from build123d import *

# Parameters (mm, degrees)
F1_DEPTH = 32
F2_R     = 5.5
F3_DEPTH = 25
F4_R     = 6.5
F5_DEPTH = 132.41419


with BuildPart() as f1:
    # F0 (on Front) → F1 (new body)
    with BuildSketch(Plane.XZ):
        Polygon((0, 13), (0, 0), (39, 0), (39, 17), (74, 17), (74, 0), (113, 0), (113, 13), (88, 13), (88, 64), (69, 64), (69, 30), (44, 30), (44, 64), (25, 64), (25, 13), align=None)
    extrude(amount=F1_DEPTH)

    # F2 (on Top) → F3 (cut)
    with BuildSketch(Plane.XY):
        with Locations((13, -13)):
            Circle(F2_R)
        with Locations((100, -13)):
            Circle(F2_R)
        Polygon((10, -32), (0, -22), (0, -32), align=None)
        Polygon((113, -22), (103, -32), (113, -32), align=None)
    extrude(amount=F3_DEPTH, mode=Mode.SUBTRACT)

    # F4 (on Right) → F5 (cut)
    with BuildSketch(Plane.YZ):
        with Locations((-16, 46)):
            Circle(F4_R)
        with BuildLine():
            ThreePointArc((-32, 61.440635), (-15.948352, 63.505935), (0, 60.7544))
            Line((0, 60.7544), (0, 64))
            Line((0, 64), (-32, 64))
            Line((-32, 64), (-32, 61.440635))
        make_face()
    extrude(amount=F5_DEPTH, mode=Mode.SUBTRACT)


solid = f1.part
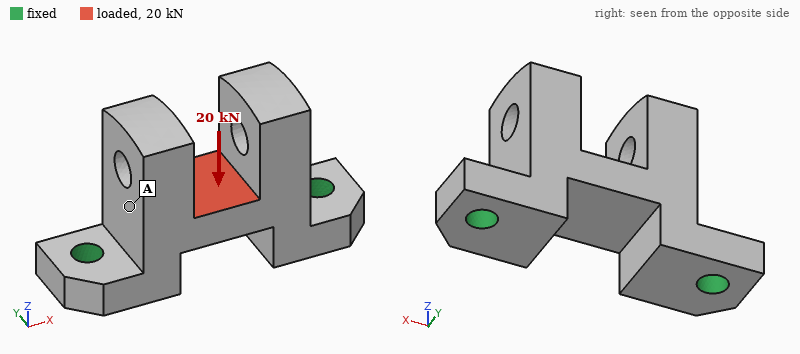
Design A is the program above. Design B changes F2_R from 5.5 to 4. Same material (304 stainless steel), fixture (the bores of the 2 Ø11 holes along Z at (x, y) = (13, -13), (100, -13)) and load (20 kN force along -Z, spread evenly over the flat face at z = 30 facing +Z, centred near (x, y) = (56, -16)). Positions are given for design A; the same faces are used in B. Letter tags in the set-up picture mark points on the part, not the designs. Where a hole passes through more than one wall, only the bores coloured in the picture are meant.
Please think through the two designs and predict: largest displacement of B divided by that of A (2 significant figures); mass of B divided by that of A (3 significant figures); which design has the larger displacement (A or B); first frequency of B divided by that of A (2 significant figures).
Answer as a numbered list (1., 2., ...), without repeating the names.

1. 1.1
2. 1.01
3. B
4. 0.90
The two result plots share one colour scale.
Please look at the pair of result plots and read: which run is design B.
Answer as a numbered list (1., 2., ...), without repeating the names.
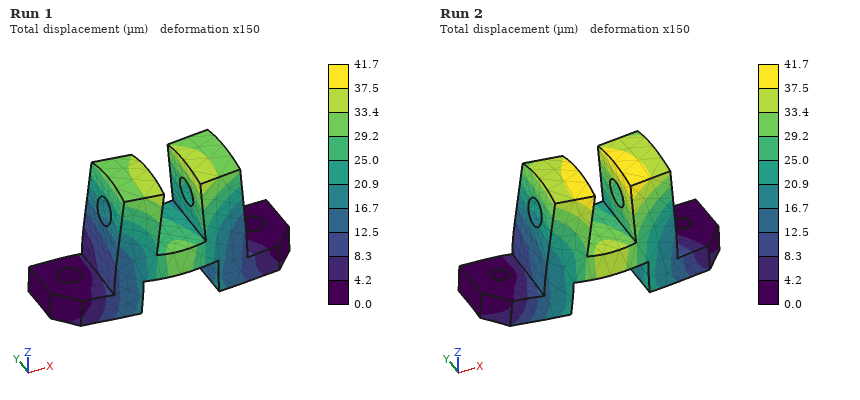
1. Run 2
